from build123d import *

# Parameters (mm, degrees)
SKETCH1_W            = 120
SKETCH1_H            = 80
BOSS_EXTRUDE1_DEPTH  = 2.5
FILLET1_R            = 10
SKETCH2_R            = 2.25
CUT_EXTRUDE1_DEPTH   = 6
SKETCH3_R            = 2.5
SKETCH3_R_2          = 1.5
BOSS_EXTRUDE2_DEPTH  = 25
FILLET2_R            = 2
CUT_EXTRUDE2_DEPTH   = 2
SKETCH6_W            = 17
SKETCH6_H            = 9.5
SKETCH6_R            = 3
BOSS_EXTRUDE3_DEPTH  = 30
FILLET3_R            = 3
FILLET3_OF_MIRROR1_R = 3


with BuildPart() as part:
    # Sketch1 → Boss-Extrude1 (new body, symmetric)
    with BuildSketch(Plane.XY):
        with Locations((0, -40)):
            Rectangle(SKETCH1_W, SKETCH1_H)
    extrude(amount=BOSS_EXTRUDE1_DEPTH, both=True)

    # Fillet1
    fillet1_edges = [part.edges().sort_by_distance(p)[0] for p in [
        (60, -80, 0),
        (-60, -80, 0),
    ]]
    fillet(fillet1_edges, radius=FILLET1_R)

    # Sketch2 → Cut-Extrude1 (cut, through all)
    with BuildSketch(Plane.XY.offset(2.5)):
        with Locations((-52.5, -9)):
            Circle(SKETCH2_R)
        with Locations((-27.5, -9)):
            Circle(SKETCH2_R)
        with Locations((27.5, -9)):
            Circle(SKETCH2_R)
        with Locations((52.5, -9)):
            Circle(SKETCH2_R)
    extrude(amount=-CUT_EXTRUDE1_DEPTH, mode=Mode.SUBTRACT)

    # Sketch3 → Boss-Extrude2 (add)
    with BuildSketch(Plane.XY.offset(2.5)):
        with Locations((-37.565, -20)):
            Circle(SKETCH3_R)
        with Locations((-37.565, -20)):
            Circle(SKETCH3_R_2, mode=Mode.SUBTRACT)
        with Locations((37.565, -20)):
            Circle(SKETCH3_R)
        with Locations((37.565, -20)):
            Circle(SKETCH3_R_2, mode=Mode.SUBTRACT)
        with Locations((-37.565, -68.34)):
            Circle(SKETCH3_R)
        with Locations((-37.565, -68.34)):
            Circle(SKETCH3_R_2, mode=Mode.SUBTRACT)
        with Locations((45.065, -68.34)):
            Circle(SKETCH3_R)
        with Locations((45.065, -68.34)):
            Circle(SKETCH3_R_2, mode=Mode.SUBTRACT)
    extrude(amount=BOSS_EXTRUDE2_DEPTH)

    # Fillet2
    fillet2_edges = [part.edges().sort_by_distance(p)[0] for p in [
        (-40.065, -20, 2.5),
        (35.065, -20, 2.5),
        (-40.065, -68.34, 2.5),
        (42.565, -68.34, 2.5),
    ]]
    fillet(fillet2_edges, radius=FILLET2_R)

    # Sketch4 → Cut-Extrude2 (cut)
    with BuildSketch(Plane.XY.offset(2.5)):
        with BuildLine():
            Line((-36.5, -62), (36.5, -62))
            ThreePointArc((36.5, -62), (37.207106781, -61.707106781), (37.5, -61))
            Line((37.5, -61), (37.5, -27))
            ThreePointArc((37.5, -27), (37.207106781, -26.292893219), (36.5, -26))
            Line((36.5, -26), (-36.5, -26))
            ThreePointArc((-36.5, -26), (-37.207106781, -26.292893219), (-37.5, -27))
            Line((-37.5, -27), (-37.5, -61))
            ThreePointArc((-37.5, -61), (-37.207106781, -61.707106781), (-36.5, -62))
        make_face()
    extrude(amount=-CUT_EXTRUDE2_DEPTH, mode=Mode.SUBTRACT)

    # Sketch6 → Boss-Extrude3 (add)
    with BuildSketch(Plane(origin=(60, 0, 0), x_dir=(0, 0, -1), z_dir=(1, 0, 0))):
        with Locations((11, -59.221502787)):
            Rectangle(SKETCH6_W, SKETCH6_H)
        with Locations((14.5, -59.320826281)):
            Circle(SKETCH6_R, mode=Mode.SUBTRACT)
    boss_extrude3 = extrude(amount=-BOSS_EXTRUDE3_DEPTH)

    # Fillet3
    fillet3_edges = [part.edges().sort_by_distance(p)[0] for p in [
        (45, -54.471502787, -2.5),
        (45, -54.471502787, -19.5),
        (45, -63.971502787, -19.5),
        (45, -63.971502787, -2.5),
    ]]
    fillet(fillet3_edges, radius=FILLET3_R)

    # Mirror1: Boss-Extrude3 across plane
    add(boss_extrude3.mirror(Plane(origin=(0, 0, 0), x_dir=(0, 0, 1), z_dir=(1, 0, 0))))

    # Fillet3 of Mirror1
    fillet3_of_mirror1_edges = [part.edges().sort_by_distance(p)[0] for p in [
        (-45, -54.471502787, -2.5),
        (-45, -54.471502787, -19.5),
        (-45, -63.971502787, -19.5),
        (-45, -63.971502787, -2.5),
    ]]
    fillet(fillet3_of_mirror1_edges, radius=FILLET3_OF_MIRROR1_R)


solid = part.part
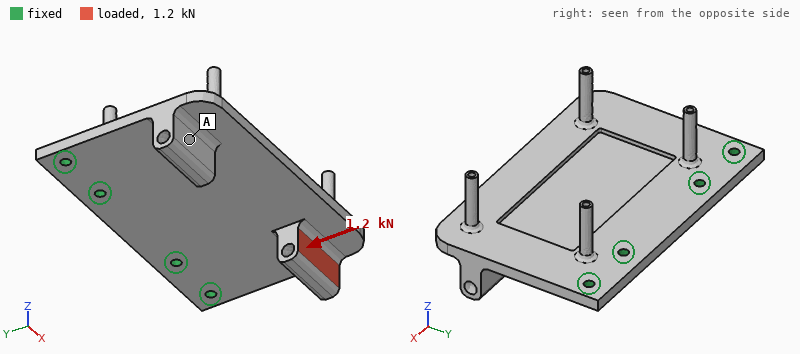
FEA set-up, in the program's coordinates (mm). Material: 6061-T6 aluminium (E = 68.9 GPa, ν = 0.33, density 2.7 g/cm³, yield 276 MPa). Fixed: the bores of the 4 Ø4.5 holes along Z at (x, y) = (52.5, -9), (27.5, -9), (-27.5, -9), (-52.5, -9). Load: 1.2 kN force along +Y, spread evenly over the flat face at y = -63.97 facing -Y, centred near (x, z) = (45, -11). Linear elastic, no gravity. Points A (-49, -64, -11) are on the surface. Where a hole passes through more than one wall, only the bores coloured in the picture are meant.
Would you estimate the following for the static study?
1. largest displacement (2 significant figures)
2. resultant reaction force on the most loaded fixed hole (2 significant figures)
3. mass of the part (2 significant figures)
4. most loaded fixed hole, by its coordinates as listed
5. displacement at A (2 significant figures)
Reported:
0.72 mm
770 N
140 g
(27.5, -9)
0.19 mm
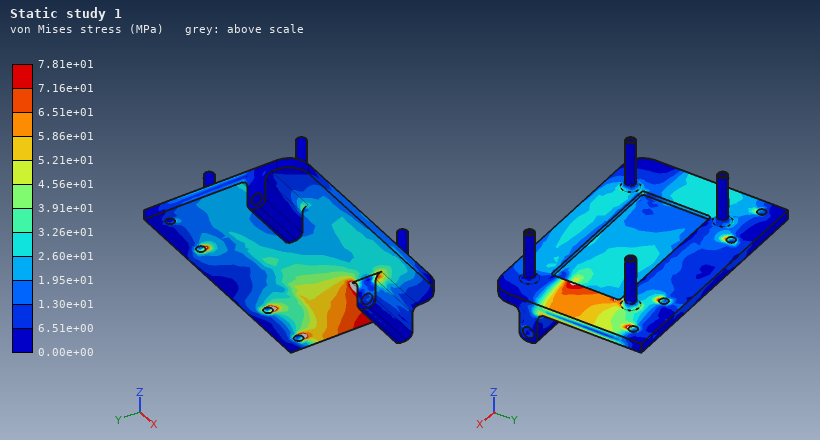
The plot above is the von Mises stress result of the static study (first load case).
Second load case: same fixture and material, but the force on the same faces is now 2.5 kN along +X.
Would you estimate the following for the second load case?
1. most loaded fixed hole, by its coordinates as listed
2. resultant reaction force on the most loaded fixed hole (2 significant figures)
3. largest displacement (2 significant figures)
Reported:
(52.5, -9)
1.6 kN
0.52 mm
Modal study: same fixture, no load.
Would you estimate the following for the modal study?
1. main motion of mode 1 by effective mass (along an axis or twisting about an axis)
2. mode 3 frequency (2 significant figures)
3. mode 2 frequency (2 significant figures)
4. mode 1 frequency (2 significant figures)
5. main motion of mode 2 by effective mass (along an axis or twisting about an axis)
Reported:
along Z
2200 Hz
1000 Hz
610 Hz
twisting about Y
